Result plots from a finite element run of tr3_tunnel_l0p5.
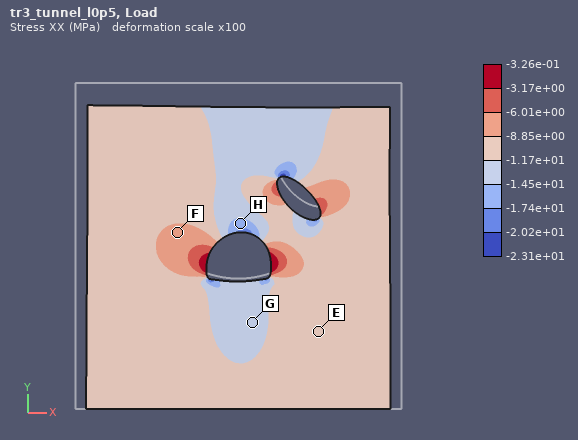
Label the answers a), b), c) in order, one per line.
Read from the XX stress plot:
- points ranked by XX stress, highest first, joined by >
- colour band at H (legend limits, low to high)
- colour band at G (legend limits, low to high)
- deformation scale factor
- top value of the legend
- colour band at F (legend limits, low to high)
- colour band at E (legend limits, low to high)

a) F > E > G > H
b) -1.74e+01 to -1.45e+01 MPa
c) -1.45e+01 to -1.17e+01 MPa
d) 100
e) -3.26e-01 MPa
f) -8.85e+00 to -6.01e+00 MPa
g) -1.17e+01 to -8.85e+00 MPa
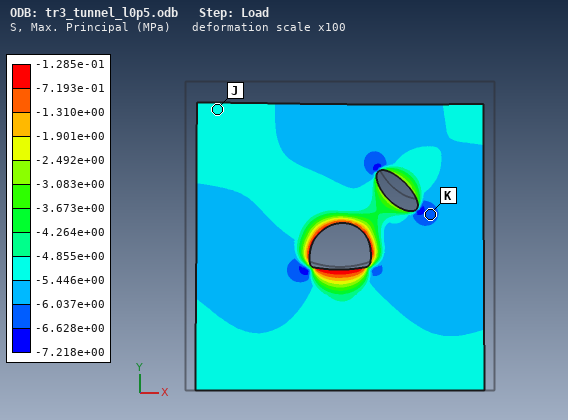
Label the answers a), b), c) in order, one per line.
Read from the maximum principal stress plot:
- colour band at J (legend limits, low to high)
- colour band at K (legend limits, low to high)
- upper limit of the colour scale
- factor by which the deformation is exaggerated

a) -5.446e+00 to -4.855e+00 MPa
b) -6.628e+00 to -6.037e+00 MPa
c) -1.285e-01 MPa
d) 100
